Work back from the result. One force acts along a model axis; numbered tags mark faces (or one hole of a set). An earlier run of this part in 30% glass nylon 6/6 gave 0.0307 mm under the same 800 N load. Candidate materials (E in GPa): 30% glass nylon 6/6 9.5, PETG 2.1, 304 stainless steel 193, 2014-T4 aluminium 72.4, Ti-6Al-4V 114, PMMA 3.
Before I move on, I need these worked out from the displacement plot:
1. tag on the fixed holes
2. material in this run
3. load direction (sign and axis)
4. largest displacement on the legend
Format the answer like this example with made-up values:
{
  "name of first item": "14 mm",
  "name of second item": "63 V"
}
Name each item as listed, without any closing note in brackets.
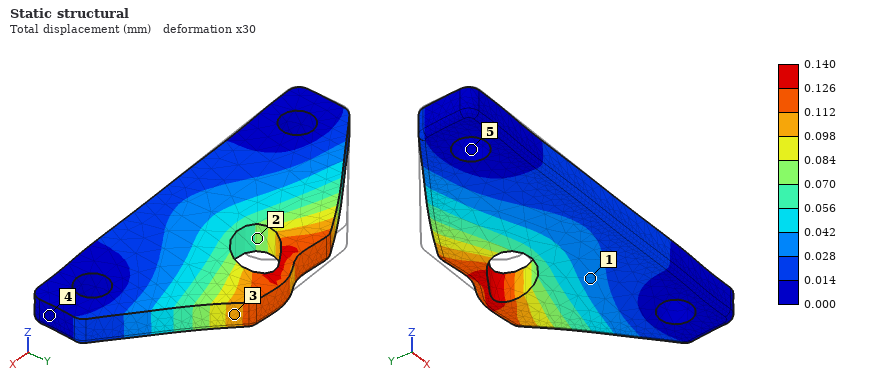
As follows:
{
  "tag on the fixed holes": "5",
  "material in this run": "PETG",
  "load direction": "+X",
  "largest displacement on the legend": "0.140 mm"
}
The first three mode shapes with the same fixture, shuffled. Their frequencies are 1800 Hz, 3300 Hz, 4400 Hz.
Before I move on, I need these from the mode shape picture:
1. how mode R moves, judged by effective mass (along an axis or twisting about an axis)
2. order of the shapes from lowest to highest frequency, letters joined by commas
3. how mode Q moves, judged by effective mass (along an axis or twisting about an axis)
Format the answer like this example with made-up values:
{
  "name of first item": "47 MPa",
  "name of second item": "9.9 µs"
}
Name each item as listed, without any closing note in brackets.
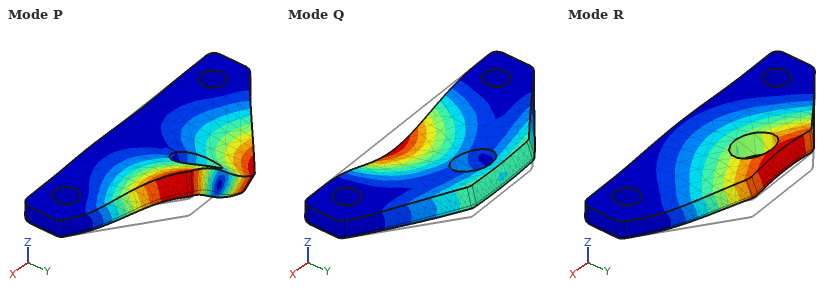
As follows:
{
  "how mode R moves, judged by effective mass": "along Z",
  "order of the shapes from lowest to highest frequency, letters joined by commas": "R, Q, P",
  "how mode Q moves, judged by effective mass": "along Z"
}
